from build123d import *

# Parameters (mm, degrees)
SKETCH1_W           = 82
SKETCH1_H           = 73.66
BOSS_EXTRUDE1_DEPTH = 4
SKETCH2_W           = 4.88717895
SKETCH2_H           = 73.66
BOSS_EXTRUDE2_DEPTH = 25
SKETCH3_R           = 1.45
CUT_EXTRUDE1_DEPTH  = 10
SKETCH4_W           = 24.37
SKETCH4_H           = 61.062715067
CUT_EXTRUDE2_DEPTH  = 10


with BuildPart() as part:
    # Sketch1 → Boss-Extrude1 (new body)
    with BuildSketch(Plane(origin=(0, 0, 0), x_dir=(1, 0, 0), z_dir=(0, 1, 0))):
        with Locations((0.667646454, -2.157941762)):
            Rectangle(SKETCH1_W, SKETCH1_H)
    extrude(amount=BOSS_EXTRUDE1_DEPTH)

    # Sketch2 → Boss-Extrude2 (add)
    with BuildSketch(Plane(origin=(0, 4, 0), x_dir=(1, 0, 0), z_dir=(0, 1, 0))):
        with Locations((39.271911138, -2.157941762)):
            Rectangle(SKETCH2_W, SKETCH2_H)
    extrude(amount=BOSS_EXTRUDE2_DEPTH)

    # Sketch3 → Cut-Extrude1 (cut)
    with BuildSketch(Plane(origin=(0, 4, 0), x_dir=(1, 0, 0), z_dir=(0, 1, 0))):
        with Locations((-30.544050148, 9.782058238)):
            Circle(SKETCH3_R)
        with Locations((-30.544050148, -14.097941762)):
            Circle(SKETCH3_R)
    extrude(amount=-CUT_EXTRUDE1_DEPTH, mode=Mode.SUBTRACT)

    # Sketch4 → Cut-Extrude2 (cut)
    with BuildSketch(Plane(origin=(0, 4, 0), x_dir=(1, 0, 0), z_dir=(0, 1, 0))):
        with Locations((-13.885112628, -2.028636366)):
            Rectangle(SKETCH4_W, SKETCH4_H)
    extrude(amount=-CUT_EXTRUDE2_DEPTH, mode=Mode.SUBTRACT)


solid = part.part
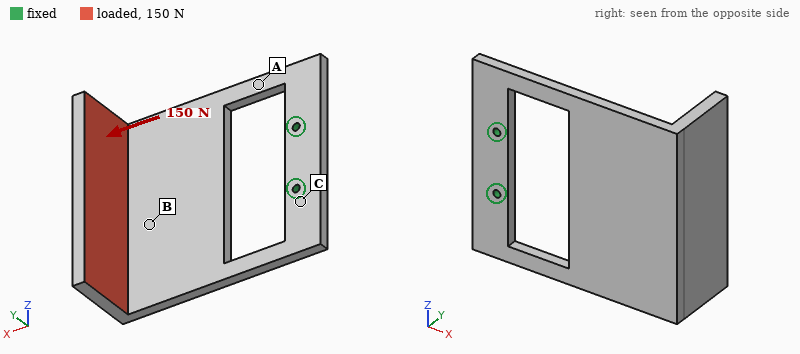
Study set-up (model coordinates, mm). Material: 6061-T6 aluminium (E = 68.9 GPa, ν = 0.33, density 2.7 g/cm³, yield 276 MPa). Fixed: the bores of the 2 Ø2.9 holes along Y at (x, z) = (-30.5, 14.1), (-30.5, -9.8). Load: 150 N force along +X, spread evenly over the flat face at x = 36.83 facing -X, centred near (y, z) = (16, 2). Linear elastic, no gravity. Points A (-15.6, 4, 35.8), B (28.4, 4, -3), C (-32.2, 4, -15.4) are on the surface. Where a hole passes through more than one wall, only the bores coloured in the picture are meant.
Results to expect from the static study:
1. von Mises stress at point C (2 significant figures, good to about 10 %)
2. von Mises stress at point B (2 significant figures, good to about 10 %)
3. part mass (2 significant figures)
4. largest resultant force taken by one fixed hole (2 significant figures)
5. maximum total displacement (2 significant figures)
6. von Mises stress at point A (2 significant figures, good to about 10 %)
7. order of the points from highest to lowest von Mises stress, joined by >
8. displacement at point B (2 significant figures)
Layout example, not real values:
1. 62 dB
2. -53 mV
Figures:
1. 30 MPa
2. 9.7 MPa
3. 73 g
4. 120 N
5. 1.3 mm
6. 67 MPa
7. A > C > B
8. 0.88 mm
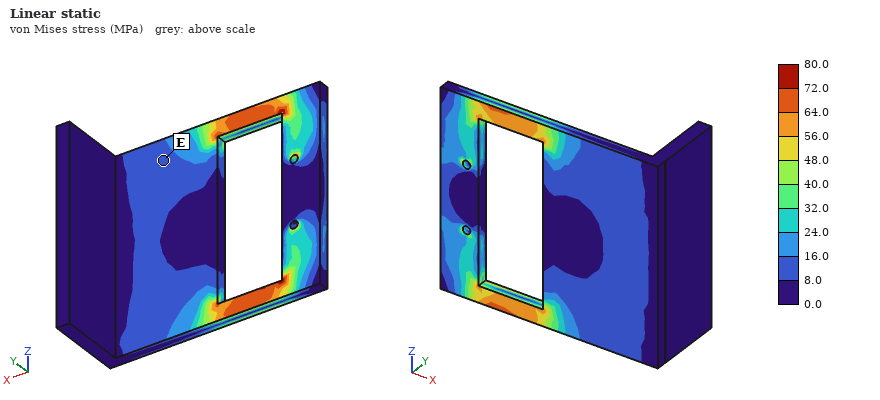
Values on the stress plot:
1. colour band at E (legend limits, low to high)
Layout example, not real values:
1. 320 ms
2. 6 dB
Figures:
1. 8.0 to 16.0 MPa
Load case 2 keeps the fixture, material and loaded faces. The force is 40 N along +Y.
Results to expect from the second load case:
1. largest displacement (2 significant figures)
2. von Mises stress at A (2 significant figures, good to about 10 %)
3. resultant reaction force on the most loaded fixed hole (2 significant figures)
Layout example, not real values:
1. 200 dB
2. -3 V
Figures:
1. 1.3 mm
2. 62 MPa
3. 20 N
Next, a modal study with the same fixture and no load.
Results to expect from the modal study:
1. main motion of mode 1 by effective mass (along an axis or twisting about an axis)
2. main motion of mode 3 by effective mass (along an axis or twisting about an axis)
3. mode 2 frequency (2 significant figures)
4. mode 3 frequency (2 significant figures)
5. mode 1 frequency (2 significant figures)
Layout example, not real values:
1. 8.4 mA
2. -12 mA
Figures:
1. along Y
2. along Z
3. 560 Hz
4. 930 Hz
5. 140 Hz
